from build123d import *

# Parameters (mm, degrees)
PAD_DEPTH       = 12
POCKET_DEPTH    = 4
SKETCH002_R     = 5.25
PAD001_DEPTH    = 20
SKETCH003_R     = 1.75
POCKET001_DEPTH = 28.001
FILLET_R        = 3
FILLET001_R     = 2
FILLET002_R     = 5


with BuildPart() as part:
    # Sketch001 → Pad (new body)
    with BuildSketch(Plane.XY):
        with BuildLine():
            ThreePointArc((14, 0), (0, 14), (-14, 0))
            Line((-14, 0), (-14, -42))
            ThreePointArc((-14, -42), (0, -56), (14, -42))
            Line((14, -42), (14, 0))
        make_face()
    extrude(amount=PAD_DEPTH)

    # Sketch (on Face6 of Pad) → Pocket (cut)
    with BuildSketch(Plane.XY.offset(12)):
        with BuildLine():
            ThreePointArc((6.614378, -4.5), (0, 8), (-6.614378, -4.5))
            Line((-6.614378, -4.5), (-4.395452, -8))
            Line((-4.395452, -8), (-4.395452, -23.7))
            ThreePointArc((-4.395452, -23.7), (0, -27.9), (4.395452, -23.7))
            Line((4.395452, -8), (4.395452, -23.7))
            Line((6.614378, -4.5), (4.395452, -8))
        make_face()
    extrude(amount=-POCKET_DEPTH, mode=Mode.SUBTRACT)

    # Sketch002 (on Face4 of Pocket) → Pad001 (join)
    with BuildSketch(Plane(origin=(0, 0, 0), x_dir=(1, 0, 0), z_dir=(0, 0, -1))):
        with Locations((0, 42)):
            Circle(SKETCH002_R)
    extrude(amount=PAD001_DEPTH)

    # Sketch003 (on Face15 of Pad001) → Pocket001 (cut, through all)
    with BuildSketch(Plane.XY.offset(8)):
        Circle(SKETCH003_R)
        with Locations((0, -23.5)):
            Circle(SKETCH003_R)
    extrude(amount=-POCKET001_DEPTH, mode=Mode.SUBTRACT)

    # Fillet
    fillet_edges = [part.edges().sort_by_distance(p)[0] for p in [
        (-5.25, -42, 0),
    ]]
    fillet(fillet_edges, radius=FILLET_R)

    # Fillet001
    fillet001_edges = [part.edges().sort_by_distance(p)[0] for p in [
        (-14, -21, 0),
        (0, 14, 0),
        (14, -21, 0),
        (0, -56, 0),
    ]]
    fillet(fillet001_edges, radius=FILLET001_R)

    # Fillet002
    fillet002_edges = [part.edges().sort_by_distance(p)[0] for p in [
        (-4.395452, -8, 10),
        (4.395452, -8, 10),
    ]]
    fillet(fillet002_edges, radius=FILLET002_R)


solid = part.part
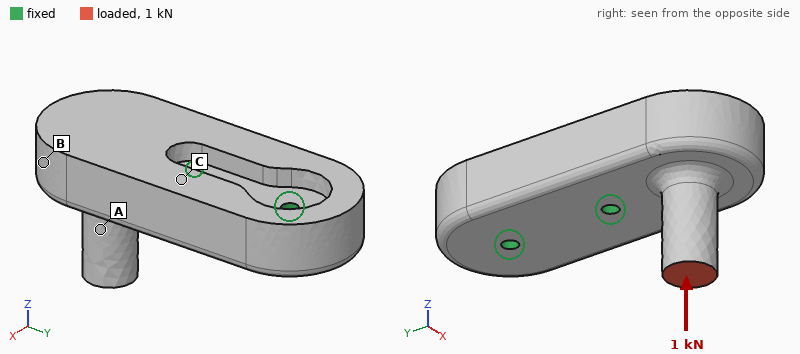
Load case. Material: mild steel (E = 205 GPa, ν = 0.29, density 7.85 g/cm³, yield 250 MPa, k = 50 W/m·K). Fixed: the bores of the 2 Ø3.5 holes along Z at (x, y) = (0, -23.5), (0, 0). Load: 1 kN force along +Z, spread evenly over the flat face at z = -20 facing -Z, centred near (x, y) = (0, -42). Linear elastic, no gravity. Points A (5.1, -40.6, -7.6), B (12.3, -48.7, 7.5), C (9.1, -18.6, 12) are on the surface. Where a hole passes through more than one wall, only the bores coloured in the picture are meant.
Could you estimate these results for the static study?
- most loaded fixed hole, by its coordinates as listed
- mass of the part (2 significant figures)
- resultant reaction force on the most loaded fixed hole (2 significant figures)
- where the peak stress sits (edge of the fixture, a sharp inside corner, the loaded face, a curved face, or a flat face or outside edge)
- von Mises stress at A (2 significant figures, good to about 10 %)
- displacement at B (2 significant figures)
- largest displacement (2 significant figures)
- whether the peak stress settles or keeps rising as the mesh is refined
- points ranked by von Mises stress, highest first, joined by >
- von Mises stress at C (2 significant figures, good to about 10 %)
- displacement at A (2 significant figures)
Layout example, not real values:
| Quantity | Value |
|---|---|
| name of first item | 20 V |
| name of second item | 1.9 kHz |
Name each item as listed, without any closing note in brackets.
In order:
| Quantity | Value |
|---|---|
| most loaded fixed hole, by its coordinates as listed | (0, -23.5) |
| mass of the part | 170 g |
| resultant reaction force on the most loaded fixed hole | 1.5 kN |
| where the peak stress sits | edge of the fixture |
| von Mises stress at A | 11 MPa |
| displacement at B | 9.7 µm |
| largest displacement | 15 µm |
| whether the peak stress settles or keeps rising as the mesh is refined | keeps rising |
| points ranked by von Mises stress, highest first, joined by > | C > A > B |
| von Mises stress at C | 19 MPa |
| displacement at A | 8.7 µm |
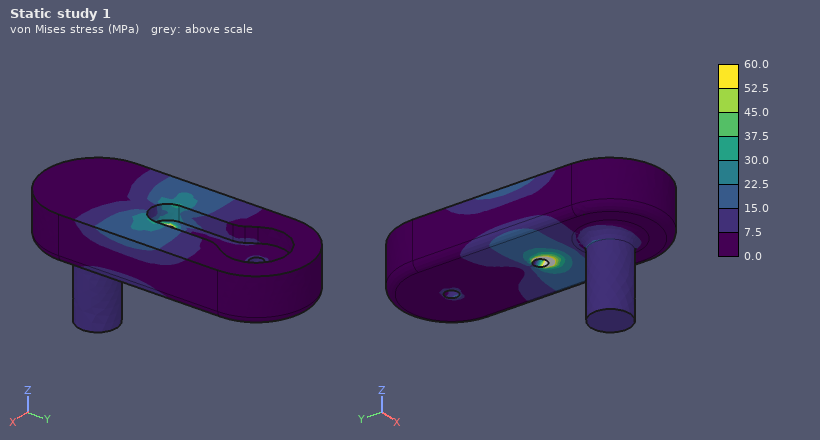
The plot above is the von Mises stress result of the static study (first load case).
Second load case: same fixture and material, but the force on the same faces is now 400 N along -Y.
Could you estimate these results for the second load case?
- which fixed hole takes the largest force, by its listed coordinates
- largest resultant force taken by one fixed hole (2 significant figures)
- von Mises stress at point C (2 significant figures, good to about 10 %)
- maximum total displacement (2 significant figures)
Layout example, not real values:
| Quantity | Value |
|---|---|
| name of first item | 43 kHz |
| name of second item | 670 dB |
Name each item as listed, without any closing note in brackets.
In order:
| Quantity | Value |
|---|---|
| which fixed hole takes the largest force, by its listed coordinates | (0, -23.5) |
| largest resultant force taken by one fixed hole | 560 N |
| von Mises stress at point C | 9.8 MPa |
| maximum total displacement | 21 µm |
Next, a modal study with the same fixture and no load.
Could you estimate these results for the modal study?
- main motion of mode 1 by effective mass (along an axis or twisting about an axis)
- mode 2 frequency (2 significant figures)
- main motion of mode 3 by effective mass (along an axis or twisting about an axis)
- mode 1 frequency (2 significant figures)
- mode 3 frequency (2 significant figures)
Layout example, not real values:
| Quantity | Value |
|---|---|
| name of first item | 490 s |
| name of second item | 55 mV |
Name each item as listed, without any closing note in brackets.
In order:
| Quantity | Value |
|---|---|
| main motion of mode 1 by effective mass | along Z |
| mode 2 frequency | 8300 Hz |
| main motion of mode 3 by effective mass | along X |
| mode 1 frequency | 6000 Hz |
| mode 3 frequency | 10 kHz |
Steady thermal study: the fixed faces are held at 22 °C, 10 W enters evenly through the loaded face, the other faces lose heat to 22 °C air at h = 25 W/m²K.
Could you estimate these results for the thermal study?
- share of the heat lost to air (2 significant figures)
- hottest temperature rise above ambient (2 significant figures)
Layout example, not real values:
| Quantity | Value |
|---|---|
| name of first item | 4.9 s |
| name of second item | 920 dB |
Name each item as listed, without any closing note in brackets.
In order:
| Quantity | Value |
|---|---|
| share of the heat lost to air | 13 % |
| hottest temperature rise above ambient | 60 K |
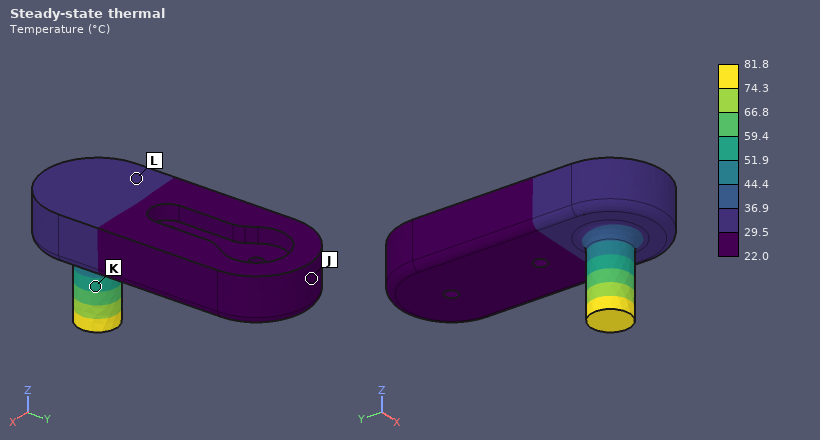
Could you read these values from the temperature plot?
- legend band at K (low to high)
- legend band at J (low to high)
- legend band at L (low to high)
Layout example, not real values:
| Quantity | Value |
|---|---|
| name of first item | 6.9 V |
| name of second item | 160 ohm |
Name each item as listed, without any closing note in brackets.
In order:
| Quantity | Value |
|---|---|
| legend band at K | 51.9 to 59.4 °C |
| legend band at J | 22.0 to 29.5 °C |
| legend band at L | 29.5 to 36.9 °C |
